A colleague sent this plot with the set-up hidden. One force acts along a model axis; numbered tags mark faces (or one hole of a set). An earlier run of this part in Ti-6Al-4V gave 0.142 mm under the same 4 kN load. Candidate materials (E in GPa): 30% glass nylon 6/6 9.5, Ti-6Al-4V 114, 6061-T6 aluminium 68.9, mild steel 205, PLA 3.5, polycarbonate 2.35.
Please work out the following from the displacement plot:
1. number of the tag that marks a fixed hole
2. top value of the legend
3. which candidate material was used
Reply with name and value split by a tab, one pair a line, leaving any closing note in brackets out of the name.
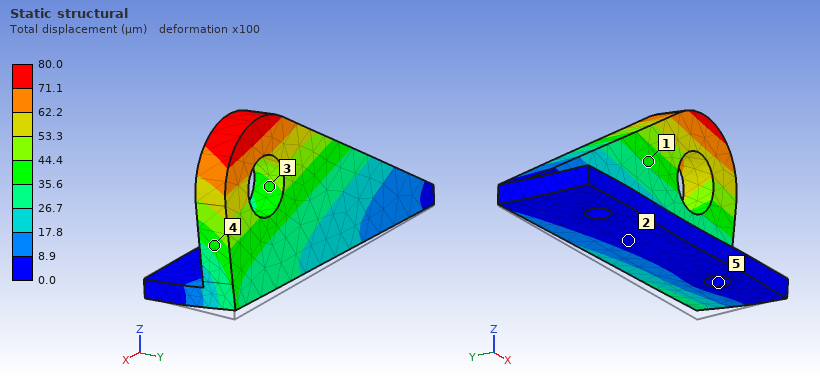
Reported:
number of the tag that marks a fixed hole	5
top value of the legend	80.0 µm
which candidate material was used	mild steel
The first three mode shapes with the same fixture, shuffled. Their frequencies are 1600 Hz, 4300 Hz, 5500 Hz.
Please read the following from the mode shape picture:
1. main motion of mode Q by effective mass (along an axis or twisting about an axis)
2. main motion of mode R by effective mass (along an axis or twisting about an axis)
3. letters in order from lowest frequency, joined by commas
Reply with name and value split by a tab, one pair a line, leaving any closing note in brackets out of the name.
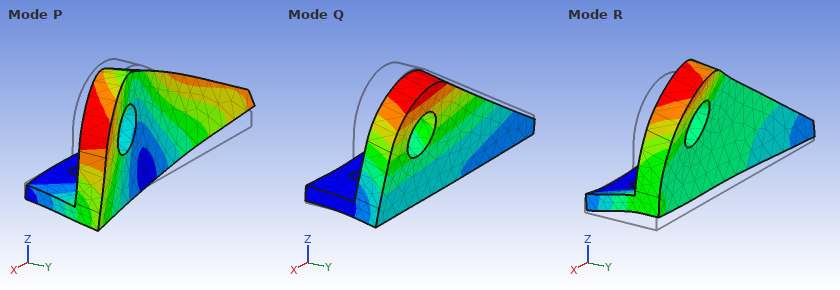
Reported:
main motion of mode Q by effective mass	along Y
main motion of mode R by effective mass	along Z
letters in order from lowest frequency, joined by commas	Q, P, R
